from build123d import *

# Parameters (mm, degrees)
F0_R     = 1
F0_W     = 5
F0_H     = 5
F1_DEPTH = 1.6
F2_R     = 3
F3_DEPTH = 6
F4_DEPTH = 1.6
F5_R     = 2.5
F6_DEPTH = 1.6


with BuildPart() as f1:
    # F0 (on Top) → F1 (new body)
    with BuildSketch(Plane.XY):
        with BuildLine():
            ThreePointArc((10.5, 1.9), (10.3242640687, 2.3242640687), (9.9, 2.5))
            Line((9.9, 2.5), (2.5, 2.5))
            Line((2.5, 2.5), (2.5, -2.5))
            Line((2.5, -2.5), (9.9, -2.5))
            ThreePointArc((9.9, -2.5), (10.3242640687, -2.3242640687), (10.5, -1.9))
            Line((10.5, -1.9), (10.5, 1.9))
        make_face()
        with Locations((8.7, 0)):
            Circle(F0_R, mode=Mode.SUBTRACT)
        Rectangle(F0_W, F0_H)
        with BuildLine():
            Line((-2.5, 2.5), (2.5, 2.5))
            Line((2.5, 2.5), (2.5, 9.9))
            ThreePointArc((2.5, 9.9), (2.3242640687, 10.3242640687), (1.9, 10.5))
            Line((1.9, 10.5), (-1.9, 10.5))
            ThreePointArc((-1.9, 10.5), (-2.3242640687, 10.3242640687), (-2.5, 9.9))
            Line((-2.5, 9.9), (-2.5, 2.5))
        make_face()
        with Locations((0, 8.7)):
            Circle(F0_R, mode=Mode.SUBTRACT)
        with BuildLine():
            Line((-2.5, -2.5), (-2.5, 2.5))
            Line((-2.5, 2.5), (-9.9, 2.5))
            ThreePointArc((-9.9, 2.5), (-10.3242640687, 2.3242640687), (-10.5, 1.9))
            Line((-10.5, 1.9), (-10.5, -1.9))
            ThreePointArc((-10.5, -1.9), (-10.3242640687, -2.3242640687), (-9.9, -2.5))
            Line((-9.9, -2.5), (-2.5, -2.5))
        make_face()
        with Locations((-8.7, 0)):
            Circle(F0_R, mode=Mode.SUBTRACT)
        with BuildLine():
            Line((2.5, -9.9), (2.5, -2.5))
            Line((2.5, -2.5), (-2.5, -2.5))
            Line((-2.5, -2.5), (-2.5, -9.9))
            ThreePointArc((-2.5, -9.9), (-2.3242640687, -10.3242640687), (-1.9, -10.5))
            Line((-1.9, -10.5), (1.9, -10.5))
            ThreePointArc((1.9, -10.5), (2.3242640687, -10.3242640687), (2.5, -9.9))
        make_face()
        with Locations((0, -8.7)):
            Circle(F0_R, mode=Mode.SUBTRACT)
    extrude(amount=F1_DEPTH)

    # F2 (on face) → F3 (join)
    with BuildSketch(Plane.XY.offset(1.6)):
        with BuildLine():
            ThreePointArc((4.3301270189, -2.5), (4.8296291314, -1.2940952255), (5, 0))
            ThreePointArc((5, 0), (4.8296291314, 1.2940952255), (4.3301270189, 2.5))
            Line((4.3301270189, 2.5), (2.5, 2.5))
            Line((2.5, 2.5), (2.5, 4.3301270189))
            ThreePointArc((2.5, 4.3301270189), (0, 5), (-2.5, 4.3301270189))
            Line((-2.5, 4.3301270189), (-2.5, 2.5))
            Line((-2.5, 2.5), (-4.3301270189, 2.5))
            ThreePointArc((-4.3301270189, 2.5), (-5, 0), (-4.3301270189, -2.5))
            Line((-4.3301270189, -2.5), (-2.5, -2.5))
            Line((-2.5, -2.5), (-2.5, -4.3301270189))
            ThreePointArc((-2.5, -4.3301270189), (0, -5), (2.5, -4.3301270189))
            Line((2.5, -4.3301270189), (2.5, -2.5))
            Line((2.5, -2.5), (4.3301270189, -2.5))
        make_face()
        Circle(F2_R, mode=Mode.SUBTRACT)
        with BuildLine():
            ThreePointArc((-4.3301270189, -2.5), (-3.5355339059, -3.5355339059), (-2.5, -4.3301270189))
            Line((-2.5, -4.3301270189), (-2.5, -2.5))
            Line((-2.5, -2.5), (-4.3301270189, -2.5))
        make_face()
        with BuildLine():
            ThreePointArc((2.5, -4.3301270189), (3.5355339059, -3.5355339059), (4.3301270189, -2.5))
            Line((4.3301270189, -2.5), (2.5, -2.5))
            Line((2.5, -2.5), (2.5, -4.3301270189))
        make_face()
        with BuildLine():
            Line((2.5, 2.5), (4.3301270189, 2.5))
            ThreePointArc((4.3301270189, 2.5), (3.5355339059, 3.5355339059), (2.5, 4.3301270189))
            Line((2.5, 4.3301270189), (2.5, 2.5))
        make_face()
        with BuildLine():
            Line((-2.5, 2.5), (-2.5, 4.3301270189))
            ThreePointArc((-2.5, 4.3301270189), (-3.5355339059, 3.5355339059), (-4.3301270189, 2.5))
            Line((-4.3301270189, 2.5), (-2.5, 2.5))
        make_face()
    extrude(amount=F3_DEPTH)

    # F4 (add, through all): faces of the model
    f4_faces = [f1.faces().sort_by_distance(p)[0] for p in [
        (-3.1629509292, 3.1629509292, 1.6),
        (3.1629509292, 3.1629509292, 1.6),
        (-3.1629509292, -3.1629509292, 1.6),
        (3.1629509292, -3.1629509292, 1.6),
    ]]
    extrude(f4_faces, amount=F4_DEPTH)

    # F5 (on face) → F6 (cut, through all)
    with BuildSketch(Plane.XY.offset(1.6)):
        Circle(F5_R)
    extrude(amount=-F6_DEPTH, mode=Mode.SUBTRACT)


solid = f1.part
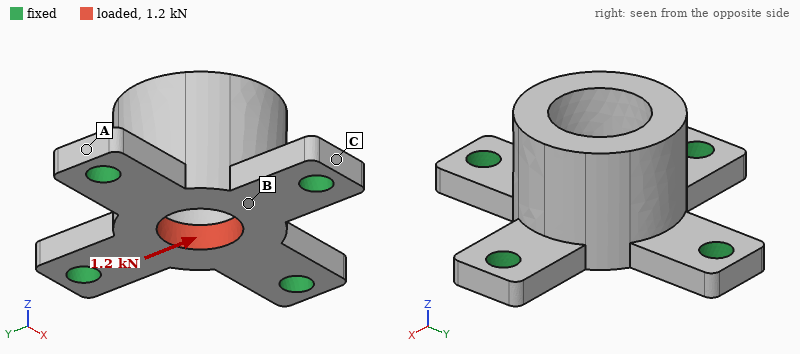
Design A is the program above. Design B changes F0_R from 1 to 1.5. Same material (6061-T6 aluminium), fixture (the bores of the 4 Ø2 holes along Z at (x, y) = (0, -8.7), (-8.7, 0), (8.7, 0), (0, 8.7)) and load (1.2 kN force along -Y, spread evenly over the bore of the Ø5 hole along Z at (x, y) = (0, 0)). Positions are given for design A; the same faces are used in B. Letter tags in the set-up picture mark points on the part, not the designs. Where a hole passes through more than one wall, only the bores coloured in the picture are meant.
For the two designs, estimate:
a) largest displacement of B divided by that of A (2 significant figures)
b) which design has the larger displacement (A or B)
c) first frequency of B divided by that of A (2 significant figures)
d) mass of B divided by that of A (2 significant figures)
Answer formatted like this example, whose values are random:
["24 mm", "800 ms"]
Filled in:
["0.85", "A", "1.1", "0.95"]
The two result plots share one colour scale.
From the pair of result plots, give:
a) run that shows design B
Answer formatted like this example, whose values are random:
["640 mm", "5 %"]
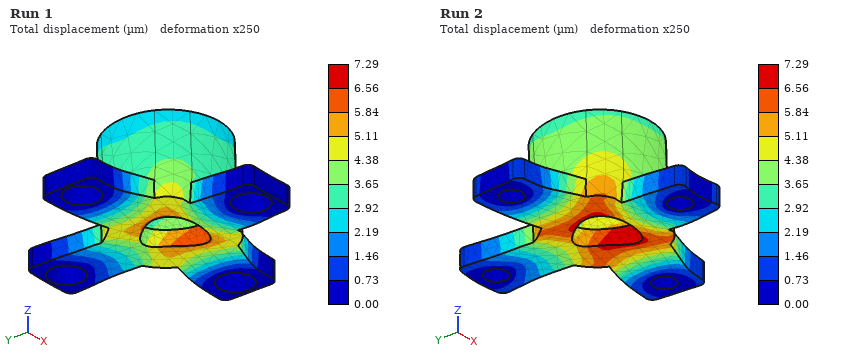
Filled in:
["Run 1"]
